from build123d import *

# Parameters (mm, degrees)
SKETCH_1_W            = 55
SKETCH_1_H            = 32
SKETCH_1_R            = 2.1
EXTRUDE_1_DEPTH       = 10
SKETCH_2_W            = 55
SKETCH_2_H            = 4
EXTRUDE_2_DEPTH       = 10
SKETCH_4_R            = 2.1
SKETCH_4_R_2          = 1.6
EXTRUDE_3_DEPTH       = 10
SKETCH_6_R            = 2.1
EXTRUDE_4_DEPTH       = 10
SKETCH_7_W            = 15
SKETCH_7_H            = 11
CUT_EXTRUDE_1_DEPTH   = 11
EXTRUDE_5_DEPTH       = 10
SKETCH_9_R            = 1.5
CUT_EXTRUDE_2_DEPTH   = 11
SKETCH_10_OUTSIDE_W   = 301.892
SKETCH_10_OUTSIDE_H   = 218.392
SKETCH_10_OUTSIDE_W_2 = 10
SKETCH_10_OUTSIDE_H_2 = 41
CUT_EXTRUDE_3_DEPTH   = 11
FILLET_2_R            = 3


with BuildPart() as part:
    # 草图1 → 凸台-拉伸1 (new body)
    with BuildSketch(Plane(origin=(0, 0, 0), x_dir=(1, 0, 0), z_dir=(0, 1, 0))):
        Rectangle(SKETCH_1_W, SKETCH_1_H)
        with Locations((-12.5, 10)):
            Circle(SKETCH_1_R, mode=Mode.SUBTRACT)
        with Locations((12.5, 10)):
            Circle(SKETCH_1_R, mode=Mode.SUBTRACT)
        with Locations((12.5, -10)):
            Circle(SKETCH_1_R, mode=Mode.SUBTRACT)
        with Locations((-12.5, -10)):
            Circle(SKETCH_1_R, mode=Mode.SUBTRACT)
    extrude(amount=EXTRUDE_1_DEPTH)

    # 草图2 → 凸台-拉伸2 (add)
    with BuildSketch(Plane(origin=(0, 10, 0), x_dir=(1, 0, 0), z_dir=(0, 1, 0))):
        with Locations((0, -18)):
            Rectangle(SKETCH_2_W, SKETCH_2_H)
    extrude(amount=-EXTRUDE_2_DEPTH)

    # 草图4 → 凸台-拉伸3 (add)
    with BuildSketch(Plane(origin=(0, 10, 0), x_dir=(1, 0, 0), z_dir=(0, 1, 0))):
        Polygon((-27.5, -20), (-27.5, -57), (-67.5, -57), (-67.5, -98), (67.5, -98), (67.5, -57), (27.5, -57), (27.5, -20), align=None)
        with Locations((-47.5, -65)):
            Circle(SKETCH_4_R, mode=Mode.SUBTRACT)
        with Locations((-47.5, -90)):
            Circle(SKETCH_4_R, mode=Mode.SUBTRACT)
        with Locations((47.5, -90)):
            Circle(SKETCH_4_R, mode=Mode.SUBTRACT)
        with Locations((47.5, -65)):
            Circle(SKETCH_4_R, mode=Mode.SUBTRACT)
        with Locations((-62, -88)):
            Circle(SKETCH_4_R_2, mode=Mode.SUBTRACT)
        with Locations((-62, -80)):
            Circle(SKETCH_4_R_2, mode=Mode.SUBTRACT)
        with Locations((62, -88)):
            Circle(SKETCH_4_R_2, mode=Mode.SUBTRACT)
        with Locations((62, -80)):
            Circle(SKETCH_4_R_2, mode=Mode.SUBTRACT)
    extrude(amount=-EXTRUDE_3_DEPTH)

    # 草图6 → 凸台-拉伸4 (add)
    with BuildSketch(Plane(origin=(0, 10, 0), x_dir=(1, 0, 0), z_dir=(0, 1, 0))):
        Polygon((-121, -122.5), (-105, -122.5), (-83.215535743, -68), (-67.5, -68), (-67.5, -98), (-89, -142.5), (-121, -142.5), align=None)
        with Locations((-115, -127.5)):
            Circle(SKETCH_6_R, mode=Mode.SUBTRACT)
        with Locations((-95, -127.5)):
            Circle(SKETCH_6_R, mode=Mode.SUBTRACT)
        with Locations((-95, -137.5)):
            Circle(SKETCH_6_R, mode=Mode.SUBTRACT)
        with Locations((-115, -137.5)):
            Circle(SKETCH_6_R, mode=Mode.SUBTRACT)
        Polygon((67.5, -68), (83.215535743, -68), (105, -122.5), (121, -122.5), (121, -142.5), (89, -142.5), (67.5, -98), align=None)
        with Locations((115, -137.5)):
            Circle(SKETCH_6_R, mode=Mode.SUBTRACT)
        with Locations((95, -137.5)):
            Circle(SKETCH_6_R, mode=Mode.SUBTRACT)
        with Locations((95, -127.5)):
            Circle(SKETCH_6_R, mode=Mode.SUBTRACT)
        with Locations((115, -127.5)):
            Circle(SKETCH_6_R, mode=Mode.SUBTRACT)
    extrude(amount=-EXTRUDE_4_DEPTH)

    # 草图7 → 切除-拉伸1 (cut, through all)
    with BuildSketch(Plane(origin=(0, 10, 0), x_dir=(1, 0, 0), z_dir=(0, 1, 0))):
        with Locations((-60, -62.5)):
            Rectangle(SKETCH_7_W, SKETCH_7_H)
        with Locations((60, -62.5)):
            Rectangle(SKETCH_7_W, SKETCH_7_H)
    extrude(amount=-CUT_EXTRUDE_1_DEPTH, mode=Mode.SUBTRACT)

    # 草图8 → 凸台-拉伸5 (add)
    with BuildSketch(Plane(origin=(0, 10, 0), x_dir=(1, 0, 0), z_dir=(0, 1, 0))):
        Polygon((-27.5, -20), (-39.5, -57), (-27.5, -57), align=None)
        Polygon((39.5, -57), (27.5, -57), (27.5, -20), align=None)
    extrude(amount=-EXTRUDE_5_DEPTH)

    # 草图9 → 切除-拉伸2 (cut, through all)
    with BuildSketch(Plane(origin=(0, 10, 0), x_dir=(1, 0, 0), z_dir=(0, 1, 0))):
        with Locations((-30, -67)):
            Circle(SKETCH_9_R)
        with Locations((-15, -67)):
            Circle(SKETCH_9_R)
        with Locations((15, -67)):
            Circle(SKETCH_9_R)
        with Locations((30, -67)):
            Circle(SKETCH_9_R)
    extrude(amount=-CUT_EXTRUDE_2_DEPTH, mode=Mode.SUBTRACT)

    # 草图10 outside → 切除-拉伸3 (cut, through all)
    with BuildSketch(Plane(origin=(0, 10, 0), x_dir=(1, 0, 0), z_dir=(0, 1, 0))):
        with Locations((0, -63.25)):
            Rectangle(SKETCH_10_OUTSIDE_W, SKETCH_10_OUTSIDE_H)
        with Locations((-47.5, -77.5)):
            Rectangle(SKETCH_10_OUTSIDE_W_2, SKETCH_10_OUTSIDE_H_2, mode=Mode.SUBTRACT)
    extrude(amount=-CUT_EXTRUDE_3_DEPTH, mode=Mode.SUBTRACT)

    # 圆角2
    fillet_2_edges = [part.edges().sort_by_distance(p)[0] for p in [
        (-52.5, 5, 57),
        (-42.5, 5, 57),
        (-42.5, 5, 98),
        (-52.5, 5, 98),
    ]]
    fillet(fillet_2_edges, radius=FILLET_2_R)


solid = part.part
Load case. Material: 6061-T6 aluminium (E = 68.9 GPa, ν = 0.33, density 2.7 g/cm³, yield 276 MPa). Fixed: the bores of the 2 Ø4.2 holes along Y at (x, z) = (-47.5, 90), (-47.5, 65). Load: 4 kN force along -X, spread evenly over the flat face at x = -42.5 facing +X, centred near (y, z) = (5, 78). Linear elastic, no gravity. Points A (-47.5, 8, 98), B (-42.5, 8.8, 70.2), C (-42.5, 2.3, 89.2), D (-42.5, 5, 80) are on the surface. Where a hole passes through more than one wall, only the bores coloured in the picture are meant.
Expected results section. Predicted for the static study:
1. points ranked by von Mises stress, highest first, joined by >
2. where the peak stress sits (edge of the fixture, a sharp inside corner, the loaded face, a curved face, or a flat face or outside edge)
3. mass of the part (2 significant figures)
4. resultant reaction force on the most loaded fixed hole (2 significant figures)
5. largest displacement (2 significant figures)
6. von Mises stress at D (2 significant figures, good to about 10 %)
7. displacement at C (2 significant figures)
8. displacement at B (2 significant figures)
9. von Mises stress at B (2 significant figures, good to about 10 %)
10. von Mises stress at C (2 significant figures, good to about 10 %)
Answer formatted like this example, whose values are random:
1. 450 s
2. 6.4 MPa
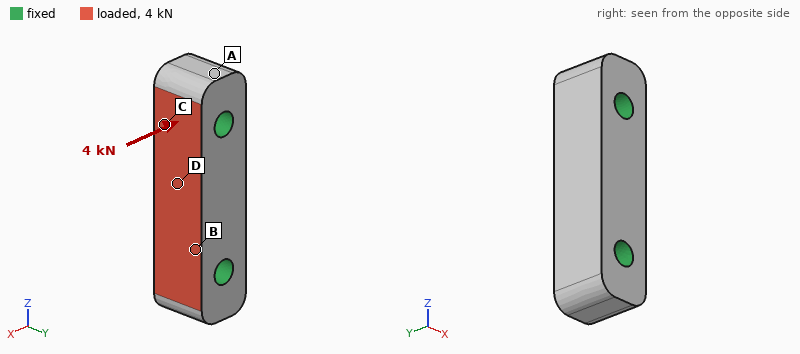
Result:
1. C > D > B > A
2. edge of the fixture
3. 10 g
4. 2.0 kN
5. 6.3 µm
6. 21 MPa
7. 1.4 µm
8. 3.8 µm
9. 10 MPa
10. 26 MPa
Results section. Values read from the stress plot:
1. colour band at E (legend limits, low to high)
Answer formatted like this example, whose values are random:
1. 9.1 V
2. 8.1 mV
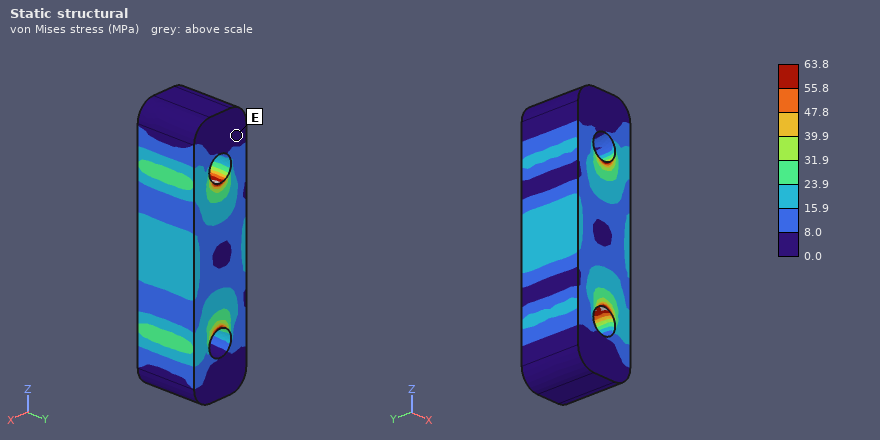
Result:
1. 0.0 to 8.0 MPa
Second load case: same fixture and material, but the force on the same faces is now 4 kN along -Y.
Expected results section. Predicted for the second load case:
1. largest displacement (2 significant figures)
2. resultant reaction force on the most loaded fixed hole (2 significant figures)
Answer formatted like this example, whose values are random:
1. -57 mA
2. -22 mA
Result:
1. 14 µm
2. 2.0 kN
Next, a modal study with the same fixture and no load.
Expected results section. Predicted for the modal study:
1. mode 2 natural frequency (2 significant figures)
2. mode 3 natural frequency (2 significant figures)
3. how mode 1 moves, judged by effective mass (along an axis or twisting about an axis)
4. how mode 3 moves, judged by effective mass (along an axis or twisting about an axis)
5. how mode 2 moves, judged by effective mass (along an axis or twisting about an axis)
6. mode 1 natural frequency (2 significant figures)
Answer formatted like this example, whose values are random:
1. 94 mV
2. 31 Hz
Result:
1. 53 kHz
2. 62 kHz
3. along X
4. twisting about Z
5. along Y
6. 47 kHz
